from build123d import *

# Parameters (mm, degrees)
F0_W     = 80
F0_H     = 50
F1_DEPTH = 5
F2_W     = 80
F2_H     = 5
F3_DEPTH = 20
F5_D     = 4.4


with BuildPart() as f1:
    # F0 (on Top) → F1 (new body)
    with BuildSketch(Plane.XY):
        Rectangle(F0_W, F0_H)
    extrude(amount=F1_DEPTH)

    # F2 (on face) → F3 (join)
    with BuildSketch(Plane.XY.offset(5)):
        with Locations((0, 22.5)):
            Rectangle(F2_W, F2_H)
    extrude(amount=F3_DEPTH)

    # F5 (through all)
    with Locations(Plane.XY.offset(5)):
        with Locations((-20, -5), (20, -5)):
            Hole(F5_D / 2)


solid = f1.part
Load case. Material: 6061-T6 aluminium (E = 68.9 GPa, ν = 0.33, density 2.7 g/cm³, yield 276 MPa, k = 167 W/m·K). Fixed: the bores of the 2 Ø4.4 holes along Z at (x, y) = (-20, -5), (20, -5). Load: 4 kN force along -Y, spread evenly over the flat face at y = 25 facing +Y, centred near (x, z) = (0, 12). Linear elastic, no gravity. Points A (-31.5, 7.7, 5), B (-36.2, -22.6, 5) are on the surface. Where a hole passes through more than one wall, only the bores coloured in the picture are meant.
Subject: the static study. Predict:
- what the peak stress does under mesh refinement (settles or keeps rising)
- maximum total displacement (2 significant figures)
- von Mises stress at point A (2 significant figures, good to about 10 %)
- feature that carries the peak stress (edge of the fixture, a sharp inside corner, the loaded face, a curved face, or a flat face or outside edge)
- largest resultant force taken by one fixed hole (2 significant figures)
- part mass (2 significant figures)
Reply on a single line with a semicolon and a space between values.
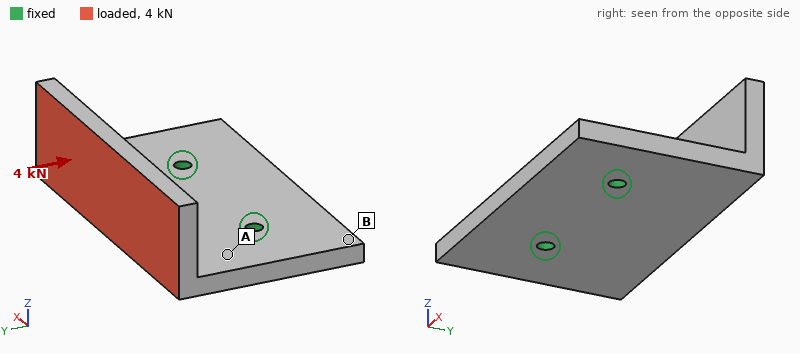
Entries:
keeps rising; 0.63 mm; 120 MPa; edge of the fixture; 2.0 kN; 75 g
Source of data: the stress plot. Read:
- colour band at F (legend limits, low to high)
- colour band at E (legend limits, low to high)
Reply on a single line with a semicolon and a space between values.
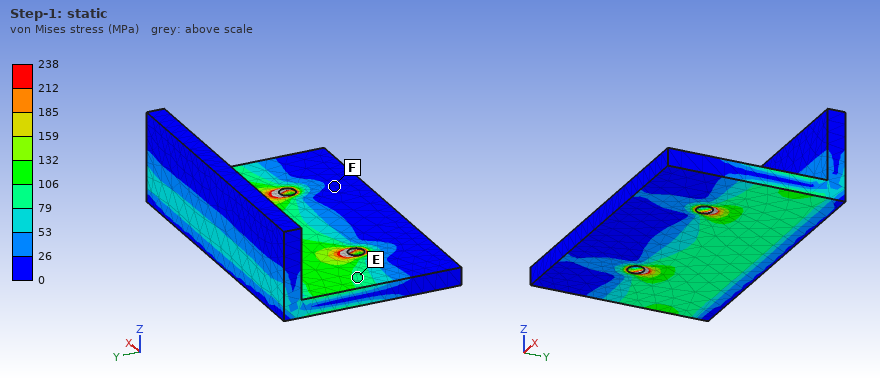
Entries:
0 to 26 MPa; 79 to 106 MPa
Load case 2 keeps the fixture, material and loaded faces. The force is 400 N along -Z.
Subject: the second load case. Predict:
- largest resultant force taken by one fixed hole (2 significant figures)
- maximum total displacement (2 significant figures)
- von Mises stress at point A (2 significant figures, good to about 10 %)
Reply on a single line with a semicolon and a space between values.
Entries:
200 N; 0.11 mm; 19 MPa
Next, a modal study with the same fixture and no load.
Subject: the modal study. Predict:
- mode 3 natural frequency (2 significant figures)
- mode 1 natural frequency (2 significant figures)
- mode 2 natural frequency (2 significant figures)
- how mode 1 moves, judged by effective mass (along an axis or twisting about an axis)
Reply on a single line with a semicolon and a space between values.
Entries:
6000 Hz; 1900 Hz; 2900 Hz; along Z
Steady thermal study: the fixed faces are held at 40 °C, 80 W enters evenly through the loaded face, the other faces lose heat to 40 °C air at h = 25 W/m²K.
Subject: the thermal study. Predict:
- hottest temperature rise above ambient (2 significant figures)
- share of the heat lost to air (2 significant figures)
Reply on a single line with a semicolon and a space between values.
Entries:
48 K; 7.4 %
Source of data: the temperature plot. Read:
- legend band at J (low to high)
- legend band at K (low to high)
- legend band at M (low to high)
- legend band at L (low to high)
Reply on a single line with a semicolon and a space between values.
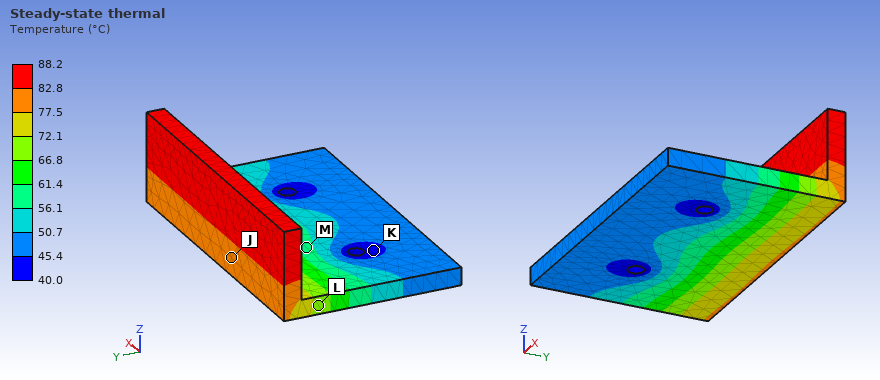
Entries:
77.5 to 82.8 °C; 40.0 to 45.4 °C; 56.1 to 61.4 °C; 66.8 to 72.1 °C
